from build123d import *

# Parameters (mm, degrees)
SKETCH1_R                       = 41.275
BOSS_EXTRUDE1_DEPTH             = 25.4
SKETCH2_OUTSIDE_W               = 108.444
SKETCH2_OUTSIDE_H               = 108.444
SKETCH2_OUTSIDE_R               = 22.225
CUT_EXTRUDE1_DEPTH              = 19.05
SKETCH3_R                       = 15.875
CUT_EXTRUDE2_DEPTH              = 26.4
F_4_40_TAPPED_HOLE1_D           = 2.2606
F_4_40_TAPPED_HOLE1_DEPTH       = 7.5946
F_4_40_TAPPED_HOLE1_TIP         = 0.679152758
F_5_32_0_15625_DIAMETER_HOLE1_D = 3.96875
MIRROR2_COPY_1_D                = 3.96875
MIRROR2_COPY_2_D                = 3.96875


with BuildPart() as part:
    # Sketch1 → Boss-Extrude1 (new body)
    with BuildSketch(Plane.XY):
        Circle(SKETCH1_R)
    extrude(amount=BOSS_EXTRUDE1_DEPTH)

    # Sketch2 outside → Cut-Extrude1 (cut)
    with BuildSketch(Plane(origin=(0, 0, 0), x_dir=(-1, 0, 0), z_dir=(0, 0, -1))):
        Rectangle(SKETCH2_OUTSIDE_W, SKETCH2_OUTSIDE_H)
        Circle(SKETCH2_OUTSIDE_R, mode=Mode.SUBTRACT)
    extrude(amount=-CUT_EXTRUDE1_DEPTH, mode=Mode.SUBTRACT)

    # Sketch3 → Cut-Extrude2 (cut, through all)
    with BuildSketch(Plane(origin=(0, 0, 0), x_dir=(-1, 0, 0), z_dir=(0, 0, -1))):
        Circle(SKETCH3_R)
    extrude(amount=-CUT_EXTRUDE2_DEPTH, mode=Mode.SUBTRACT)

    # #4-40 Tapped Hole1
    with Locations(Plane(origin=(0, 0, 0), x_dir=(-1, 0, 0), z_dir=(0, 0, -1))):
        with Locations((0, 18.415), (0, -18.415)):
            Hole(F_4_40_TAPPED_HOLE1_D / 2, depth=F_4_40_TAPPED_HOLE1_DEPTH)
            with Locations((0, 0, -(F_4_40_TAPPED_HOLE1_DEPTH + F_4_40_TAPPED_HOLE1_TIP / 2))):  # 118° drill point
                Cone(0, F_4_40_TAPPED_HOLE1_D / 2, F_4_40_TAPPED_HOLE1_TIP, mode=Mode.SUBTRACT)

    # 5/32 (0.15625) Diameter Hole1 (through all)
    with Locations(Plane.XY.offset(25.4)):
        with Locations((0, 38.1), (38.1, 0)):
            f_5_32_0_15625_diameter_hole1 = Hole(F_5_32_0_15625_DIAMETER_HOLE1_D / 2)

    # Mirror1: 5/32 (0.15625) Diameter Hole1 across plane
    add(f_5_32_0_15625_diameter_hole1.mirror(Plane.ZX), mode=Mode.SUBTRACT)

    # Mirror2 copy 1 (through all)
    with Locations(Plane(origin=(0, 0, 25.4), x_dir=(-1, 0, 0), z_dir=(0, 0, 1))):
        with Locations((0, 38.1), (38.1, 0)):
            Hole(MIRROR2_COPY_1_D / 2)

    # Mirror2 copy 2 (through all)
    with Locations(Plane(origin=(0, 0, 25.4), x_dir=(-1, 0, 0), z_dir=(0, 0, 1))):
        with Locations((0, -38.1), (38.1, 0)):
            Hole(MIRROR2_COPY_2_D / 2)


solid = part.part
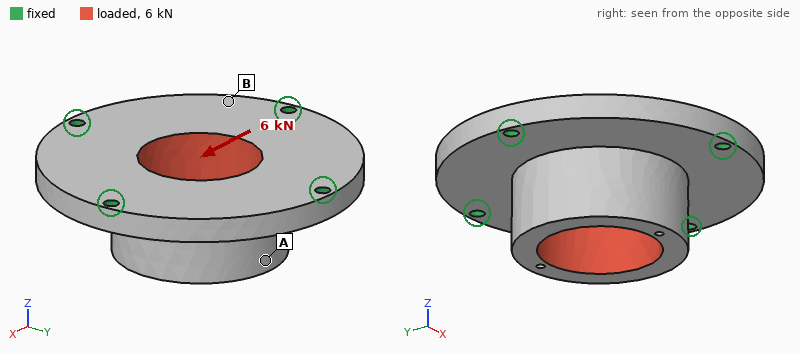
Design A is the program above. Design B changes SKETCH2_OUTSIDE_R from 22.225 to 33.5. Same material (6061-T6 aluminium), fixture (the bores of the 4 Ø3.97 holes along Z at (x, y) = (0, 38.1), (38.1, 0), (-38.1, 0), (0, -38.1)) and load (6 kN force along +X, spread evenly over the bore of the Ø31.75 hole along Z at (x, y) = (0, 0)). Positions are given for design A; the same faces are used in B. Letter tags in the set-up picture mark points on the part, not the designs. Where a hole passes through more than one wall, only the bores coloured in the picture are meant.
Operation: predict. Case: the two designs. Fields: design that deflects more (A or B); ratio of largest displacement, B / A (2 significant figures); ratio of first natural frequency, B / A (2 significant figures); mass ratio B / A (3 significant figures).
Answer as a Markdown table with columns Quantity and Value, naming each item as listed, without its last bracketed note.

| Quantity | Value |
|---|---|
| design that deflects more | A |
| ratio of largest displacement, B / A | 0.25 |
| ratio of first natural frequency, B / A | 1.3 |
| mass ratio B / A | 1.87 |
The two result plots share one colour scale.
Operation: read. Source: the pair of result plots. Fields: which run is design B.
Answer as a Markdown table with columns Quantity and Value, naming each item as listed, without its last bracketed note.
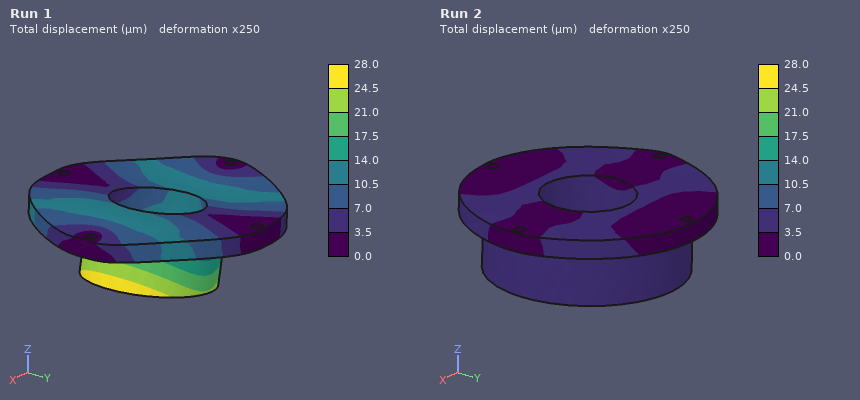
| Quantity | Value |
|---|---|
| which run is design B | Run 2 |
